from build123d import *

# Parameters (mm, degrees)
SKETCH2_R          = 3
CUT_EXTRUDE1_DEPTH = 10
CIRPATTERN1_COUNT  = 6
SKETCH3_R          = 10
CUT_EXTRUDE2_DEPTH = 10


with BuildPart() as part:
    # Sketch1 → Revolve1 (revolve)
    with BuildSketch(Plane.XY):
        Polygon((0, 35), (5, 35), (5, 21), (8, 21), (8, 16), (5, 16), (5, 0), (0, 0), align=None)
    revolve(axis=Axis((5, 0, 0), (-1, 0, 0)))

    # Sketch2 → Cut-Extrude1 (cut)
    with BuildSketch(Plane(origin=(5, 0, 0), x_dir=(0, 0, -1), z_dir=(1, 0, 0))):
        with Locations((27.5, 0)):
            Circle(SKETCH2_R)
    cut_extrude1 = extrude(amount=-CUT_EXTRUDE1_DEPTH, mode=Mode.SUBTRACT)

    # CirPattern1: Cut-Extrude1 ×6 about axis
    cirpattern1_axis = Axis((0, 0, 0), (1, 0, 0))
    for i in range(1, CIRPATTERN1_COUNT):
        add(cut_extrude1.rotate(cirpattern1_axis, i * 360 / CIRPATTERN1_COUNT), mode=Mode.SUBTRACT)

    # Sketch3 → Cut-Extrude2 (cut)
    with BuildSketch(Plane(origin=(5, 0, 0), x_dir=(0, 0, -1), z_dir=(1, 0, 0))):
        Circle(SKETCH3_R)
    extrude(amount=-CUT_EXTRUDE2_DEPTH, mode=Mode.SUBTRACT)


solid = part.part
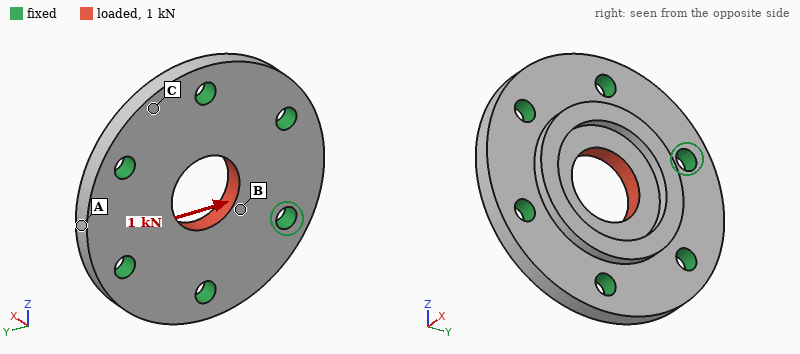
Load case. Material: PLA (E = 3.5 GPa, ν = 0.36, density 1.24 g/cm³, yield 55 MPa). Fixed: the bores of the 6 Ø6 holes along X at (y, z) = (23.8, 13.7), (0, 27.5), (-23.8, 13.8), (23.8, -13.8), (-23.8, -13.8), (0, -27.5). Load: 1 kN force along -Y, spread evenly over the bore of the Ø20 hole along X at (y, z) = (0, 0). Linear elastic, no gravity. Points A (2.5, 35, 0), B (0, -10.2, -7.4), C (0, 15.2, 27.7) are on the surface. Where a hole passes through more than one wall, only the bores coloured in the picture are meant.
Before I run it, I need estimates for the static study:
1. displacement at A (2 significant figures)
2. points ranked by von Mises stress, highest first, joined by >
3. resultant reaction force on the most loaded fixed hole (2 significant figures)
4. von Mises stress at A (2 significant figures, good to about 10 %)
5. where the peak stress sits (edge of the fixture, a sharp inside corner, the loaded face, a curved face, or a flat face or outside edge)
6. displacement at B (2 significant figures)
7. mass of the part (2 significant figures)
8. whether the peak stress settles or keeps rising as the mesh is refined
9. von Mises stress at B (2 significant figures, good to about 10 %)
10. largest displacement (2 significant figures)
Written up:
6.4 µm
B > A > C
220 N
1.4 MPa
edge of the fixture
13 µm
23 g
keeps rising
3.2 MPa
17 µm
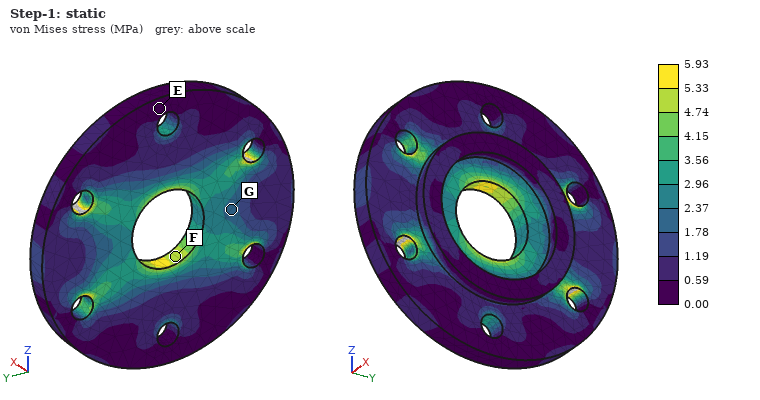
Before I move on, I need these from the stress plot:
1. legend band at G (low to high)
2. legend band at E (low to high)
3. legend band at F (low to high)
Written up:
1.78 to 2.37 MPa
0.00 to 0.59 MPa
4.74 to 5.33 MPa
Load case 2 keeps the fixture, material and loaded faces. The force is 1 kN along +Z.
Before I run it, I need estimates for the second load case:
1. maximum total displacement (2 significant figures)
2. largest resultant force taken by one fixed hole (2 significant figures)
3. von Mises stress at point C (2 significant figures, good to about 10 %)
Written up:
17 µm
250 N
0.72 MPa
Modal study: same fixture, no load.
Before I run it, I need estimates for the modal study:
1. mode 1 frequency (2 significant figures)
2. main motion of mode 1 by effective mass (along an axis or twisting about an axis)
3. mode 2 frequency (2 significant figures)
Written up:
6300 Hz
along X
8700 Hz
